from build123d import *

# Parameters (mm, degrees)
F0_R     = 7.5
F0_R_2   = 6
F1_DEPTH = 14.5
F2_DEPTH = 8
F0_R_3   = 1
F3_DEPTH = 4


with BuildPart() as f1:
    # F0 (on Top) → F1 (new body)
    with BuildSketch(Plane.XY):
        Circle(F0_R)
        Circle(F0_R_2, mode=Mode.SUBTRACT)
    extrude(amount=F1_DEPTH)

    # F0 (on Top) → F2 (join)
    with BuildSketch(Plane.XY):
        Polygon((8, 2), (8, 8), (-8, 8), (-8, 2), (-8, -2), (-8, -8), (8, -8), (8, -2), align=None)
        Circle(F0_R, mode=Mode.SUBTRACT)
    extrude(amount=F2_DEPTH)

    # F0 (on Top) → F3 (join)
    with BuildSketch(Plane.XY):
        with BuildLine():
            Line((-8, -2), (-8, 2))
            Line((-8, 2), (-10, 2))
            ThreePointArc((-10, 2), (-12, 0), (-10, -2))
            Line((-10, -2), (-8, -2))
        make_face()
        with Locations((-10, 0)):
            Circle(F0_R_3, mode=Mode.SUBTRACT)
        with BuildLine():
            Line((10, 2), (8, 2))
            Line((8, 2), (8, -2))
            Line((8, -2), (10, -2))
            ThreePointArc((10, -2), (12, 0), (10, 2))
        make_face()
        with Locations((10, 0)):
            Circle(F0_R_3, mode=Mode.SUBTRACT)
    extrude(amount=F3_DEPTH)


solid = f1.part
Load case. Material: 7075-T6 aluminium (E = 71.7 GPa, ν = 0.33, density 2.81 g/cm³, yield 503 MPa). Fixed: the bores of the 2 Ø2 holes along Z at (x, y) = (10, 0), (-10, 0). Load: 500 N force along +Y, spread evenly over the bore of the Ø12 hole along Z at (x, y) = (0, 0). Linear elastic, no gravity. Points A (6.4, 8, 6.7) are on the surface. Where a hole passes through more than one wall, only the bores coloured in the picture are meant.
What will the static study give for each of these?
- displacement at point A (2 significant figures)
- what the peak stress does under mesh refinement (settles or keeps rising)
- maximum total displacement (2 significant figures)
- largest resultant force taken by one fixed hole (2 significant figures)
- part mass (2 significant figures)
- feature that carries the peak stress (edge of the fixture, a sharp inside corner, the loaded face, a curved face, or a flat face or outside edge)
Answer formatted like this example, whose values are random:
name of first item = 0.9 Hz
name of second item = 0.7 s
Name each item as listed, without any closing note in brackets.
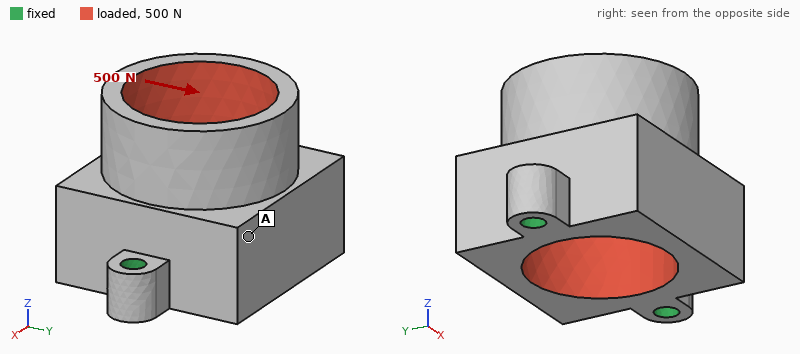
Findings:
displacement at point A = 28 µm
what the peak stress does under mesh refinement = keeps rising
maximum total displacement = 46 µm
largest resultant force taken by one fixed hole = 250 N
part mass = 4.6 g
feature that carries the peak stress = edge of the fixture
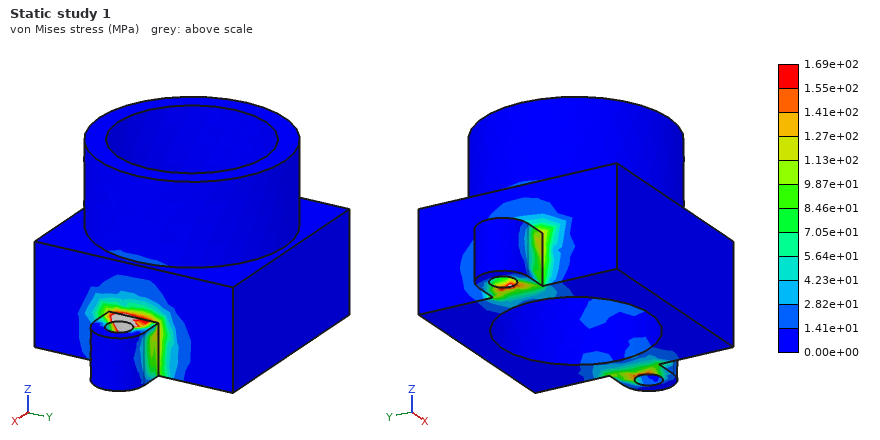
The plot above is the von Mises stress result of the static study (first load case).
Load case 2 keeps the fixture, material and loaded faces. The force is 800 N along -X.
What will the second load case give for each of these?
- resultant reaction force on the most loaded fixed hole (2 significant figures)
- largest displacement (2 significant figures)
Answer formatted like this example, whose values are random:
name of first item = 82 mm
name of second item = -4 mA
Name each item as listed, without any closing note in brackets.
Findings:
resultant reaction force on the most loaded fixed hole = 460 N
largest displacement = 8.7 µm
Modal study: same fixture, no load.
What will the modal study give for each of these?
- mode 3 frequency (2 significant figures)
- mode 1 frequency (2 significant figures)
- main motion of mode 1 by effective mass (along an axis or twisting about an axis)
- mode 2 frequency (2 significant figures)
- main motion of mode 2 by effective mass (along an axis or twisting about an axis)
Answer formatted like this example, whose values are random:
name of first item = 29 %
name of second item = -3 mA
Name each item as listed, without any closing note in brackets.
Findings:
mode 3 frequency = 27 kHz
mode 1 frequency = 9300 Hz
main motion of mode 1 by effective mass = along Y
mode 2 frequency = 26 kHz
main motion of mode 2 by effective mass = along Z
